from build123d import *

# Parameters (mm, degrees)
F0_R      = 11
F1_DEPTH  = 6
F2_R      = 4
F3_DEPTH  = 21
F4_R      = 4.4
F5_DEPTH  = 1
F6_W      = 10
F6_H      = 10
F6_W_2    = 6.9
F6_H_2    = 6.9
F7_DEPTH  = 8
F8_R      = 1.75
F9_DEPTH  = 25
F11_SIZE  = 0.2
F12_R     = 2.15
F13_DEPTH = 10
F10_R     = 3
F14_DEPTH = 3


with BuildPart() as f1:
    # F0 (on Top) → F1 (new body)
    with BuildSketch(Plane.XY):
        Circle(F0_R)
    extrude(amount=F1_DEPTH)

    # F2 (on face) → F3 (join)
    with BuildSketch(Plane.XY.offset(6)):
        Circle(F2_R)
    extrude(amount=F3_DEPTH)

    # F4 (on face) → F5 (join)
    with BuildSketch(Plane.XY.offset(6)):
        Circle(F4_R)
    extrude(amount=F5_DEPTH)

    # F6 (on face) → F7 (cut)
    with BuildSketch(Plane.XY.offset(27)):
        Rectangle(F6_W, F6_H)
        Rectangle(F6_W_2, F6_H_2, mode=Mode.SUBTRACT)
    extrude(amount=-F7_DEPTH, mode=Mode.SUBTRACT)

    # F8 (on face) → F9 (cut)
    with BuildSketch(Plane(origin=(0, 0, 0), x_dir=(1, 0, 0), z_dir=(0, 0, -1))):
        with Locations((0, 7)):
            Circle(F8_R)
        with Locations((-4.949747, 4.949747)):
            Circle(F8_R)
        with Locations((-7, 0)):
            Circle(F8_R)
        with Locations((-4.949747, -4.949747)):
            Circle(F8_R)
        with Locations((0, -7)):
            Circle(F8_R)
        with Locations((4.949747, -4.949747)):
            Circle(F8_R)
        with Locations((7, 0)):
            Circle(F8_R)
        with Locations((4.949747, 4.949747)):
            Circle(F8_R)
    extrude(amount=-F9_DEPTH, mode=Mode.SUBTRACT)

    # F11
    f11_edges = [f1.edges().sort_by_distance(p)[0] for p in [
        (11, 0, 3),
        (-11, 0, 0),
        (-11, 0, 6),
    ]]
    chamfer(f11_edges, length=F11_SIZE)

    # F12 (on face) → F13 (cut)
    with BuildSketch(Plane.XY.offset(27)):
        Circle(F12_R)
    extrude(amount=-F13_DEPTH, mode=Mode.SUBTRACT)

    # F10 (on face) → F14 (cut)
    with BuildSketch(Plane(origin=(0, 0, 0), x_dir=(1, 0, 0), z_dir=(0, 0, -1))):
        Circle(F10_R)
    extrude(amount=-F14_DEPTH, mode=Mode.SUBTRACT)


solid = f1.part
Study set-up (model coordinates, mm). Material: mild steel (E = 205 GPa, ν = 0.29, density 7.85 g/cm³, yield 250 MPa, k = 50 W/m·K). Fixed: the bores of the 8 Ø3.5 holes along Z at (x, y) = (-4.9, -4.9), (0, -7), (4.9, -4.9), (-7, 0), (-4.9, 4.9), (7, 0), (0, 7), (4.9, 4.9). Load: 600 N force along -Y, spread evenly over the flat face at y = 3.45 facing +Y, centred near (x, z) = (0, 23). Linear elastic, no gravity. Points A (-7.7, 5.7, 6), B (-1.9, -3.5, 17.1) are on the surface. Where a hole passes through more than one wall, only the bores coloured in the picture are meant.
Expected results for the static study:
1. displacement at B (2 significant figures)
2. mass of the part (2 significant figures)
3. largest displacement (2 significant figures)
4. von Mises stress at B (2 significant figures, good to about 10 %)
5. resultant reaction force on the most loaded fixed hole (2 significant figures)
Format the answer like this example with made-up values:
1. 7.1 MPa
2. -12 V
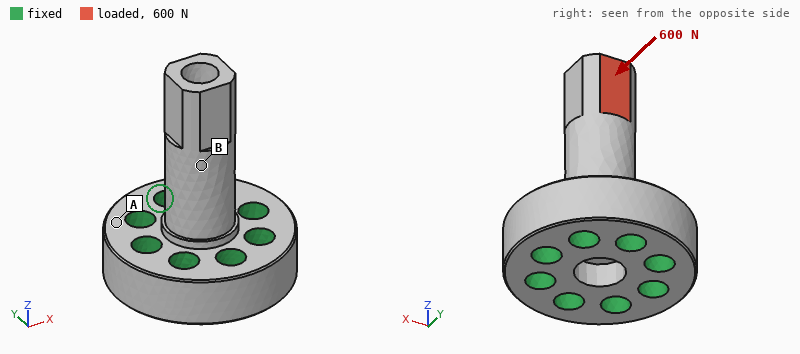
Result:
1. 18 µm
2. 20 g
3. 45 µm
4. 73 MPa
5. 580 N
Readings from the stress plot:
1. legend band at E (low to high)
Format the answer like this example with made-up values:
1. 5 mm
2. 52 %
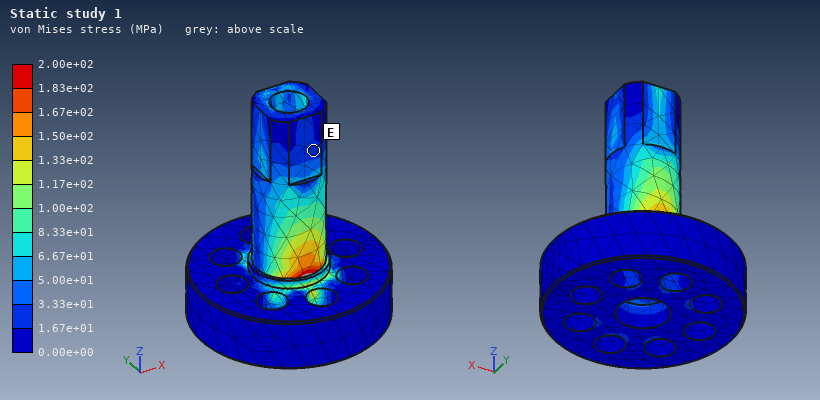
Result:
1. 1.67e+01 to 3.33e+01 MPa
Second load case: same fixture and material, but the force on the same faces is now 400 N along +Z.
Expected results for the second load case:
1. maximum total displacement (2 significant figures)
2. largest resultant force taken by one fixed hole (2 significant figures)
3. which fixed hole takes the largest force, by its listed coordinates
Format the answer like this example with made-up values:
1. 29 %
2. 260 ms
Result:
1. 9.7 µm
2. 130 N
3. (0, 7)
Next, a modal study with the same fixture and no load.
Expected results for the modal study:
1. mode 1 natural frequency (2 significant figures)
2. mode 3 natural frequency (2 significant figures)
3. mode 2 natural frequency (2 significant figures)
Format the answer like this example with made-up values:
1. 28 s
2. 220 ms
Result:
1. 14 kHz
2. 41 kHz
3. 14 kHz
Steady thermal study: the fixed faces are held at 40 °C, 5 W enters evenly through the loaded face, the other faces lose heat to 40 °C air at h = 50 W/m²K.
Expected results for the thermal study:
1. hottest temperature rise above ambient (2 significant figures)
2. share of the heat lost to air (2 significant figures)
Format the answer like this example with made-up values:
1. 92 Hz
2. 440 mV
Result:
1. 48 K
2. 16 %
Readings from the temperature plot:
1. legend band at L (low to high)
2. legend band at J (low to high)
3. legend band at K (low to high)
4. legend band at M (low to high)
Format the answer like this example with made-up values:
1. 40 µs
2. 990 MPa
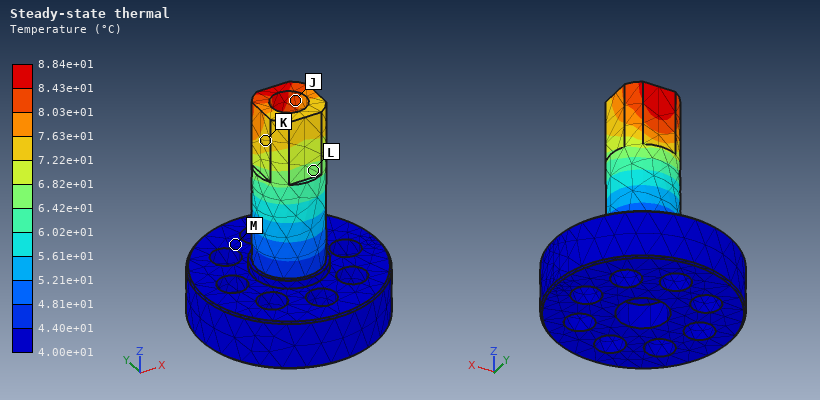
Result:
1. 6.42e+01 to 6.82e+01 °C
2. 8.03e+01 to 8.43e+01 °C
3. 7.22e+01 to 7.63e+01 °C
4. 4.00e+01 to 4.40e+01 °C
